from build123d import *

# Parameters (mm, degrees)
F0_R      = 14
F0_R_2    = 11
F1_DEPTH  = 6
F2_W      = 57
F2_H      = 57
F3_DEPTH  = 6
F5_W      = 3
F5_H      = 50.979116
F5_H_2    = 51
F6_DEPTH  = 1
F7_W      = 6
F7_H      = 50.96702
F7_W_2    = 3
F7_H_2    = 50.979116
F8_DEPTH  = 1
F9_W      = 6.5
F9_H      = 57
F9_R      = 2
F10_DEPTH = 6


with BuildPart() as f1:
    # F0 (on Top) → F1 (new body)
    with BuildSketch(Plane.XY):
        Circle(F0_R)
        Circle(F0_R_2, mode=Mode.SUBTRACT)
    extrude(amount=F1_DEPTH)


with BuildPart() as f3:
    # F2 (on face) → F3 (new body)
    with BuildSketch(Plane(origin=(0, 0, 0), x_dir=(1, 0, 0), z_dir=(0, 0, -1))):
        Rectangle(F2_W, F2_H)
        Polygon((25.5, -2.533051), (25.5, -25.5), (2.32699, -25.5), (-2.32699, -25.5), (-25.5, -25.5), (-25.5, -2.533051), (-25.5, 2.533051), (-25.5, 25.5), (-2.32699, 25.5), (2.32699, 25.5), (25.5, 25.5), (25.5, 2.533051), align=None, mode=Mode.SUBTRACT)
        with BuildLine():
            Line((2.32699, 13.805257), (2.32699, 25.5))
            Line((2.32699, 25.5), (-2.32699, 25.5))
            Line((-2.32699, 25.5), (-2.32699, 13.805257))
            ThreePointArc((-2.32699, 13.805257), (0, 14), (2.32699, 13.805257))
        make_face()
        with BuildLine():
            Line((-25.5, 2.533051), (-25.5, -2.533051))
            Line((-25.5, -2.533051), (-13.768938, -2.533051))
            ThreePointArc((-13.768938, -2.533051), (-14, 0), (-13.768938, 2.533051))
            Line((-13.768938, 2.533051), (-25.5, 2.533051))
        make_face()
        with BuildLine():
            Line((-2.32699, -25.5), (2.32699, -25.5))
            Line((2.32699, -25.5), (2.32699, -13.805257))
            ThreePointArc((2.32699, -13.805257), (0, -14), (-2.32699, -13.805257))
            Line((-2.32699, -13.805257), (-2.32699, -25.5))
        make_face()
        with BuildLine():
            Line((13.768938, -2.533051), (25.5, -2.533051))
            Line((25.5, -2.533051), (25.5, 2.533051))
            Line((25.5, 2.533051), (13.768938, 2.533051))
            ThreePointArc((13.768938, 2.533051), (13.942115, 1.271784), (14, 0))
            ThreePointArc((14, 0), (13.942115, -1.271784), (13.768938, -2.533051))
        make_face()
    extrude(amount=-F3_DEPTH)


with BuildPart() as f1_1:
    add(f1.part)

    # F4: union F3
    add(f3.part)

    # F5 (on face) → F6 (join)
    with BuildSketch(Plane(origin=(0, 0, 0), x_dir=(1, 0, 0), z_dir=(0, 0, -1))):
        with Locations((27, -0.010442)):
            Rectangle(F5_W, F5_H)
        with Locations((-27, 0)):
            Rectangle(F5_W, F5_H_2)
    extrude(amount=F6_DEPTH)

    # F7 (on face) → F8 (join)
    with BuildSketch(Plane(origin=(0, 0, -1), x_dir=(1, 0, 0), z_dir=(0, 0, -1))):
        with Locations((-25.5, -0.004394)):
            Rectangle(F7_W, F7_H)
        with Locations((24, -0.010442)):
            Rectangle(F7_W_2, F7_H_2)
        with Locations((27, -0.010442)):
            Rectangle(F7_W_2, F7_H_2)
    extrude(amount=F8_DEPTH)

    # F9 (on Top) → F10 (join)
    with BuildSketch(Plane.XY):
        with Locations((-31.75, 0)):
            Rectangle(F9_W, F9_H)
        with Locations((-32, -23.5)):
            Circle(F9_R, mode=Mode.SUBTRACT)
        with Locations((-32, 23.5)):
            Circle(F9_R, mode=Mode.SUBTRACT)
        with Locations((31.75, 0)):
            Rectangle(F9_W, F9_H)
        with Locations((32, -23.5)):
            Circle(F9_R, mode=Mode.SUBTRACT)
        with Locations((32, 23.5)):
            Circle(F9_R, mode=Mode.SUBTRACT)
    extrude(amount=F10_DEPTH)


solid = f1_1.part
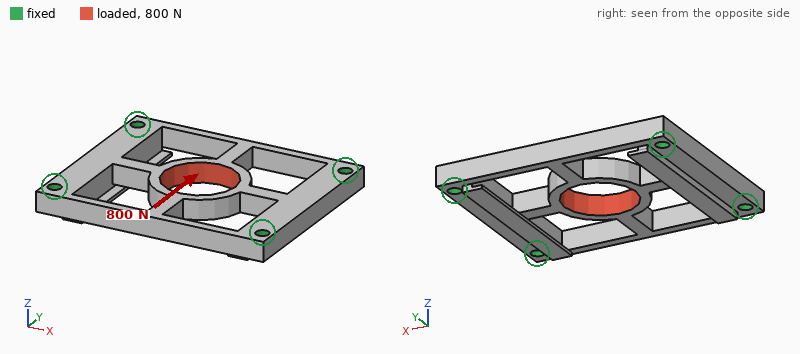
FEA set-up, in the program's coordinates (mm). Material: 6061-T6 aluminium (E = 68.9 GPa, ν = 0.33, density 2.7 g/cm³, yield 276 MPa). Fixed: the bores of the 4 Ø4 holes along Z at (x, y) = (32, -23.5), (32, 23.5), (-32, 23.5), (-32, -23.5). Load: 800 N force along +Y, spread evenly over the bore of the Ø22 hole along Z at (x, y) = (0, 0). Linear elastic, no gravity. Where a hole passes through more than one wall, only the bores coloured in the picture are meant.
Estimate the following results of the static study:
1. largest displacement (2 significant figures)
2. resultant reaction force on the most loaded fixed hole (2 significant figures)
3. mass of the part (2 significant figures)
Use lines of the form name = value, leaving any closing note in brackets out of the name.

largest displacement = 45 µm
resultant reaction force on the most loaded fixed hole = 230 N
mass of the part = 32 g
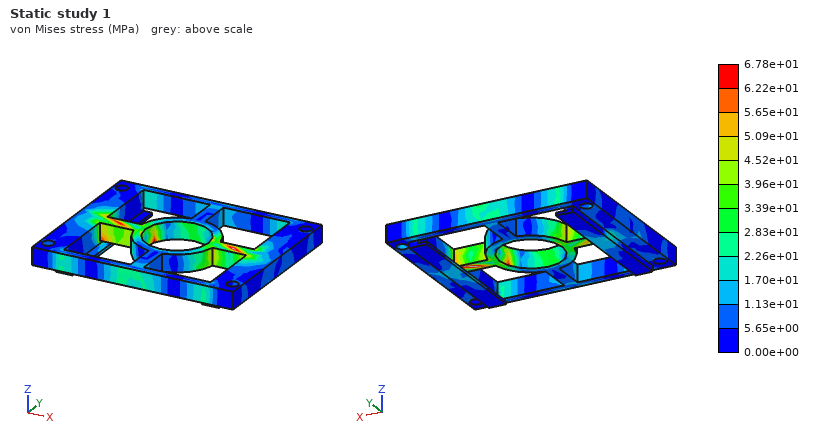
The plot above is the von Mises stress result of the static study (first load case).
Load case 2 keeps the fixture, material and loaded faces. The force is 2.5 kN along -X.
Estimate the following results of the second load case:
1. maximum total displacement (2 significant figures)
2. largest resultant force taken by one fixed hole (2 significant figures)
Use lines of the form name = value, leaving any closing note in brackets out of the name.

maximum total displacement = 69 µm
largest resultant force taken by one fixed hole = 740 N
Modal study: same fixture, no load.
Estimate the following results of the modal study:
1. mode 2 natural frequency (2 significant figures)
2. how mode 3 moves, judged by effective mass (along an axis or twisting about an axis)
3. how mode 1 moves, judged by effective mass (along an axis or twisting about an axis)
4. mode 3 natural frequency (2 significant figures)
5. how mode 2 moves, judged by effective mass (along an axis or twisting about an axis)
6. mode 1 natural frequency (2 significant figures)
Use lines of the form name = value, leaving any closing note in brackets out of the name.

mode 2 natural frequency = 7100 Hz
how mode 3 moves, judged by effective mass = along Y
how mode 1 moves, judged by effective mass = along Z
mode 3 natural frequency = 8000 Hz
how mode 2 moves, judged by effective mass = twisting about X
mode 1 natural frequency = 5500 Hz
